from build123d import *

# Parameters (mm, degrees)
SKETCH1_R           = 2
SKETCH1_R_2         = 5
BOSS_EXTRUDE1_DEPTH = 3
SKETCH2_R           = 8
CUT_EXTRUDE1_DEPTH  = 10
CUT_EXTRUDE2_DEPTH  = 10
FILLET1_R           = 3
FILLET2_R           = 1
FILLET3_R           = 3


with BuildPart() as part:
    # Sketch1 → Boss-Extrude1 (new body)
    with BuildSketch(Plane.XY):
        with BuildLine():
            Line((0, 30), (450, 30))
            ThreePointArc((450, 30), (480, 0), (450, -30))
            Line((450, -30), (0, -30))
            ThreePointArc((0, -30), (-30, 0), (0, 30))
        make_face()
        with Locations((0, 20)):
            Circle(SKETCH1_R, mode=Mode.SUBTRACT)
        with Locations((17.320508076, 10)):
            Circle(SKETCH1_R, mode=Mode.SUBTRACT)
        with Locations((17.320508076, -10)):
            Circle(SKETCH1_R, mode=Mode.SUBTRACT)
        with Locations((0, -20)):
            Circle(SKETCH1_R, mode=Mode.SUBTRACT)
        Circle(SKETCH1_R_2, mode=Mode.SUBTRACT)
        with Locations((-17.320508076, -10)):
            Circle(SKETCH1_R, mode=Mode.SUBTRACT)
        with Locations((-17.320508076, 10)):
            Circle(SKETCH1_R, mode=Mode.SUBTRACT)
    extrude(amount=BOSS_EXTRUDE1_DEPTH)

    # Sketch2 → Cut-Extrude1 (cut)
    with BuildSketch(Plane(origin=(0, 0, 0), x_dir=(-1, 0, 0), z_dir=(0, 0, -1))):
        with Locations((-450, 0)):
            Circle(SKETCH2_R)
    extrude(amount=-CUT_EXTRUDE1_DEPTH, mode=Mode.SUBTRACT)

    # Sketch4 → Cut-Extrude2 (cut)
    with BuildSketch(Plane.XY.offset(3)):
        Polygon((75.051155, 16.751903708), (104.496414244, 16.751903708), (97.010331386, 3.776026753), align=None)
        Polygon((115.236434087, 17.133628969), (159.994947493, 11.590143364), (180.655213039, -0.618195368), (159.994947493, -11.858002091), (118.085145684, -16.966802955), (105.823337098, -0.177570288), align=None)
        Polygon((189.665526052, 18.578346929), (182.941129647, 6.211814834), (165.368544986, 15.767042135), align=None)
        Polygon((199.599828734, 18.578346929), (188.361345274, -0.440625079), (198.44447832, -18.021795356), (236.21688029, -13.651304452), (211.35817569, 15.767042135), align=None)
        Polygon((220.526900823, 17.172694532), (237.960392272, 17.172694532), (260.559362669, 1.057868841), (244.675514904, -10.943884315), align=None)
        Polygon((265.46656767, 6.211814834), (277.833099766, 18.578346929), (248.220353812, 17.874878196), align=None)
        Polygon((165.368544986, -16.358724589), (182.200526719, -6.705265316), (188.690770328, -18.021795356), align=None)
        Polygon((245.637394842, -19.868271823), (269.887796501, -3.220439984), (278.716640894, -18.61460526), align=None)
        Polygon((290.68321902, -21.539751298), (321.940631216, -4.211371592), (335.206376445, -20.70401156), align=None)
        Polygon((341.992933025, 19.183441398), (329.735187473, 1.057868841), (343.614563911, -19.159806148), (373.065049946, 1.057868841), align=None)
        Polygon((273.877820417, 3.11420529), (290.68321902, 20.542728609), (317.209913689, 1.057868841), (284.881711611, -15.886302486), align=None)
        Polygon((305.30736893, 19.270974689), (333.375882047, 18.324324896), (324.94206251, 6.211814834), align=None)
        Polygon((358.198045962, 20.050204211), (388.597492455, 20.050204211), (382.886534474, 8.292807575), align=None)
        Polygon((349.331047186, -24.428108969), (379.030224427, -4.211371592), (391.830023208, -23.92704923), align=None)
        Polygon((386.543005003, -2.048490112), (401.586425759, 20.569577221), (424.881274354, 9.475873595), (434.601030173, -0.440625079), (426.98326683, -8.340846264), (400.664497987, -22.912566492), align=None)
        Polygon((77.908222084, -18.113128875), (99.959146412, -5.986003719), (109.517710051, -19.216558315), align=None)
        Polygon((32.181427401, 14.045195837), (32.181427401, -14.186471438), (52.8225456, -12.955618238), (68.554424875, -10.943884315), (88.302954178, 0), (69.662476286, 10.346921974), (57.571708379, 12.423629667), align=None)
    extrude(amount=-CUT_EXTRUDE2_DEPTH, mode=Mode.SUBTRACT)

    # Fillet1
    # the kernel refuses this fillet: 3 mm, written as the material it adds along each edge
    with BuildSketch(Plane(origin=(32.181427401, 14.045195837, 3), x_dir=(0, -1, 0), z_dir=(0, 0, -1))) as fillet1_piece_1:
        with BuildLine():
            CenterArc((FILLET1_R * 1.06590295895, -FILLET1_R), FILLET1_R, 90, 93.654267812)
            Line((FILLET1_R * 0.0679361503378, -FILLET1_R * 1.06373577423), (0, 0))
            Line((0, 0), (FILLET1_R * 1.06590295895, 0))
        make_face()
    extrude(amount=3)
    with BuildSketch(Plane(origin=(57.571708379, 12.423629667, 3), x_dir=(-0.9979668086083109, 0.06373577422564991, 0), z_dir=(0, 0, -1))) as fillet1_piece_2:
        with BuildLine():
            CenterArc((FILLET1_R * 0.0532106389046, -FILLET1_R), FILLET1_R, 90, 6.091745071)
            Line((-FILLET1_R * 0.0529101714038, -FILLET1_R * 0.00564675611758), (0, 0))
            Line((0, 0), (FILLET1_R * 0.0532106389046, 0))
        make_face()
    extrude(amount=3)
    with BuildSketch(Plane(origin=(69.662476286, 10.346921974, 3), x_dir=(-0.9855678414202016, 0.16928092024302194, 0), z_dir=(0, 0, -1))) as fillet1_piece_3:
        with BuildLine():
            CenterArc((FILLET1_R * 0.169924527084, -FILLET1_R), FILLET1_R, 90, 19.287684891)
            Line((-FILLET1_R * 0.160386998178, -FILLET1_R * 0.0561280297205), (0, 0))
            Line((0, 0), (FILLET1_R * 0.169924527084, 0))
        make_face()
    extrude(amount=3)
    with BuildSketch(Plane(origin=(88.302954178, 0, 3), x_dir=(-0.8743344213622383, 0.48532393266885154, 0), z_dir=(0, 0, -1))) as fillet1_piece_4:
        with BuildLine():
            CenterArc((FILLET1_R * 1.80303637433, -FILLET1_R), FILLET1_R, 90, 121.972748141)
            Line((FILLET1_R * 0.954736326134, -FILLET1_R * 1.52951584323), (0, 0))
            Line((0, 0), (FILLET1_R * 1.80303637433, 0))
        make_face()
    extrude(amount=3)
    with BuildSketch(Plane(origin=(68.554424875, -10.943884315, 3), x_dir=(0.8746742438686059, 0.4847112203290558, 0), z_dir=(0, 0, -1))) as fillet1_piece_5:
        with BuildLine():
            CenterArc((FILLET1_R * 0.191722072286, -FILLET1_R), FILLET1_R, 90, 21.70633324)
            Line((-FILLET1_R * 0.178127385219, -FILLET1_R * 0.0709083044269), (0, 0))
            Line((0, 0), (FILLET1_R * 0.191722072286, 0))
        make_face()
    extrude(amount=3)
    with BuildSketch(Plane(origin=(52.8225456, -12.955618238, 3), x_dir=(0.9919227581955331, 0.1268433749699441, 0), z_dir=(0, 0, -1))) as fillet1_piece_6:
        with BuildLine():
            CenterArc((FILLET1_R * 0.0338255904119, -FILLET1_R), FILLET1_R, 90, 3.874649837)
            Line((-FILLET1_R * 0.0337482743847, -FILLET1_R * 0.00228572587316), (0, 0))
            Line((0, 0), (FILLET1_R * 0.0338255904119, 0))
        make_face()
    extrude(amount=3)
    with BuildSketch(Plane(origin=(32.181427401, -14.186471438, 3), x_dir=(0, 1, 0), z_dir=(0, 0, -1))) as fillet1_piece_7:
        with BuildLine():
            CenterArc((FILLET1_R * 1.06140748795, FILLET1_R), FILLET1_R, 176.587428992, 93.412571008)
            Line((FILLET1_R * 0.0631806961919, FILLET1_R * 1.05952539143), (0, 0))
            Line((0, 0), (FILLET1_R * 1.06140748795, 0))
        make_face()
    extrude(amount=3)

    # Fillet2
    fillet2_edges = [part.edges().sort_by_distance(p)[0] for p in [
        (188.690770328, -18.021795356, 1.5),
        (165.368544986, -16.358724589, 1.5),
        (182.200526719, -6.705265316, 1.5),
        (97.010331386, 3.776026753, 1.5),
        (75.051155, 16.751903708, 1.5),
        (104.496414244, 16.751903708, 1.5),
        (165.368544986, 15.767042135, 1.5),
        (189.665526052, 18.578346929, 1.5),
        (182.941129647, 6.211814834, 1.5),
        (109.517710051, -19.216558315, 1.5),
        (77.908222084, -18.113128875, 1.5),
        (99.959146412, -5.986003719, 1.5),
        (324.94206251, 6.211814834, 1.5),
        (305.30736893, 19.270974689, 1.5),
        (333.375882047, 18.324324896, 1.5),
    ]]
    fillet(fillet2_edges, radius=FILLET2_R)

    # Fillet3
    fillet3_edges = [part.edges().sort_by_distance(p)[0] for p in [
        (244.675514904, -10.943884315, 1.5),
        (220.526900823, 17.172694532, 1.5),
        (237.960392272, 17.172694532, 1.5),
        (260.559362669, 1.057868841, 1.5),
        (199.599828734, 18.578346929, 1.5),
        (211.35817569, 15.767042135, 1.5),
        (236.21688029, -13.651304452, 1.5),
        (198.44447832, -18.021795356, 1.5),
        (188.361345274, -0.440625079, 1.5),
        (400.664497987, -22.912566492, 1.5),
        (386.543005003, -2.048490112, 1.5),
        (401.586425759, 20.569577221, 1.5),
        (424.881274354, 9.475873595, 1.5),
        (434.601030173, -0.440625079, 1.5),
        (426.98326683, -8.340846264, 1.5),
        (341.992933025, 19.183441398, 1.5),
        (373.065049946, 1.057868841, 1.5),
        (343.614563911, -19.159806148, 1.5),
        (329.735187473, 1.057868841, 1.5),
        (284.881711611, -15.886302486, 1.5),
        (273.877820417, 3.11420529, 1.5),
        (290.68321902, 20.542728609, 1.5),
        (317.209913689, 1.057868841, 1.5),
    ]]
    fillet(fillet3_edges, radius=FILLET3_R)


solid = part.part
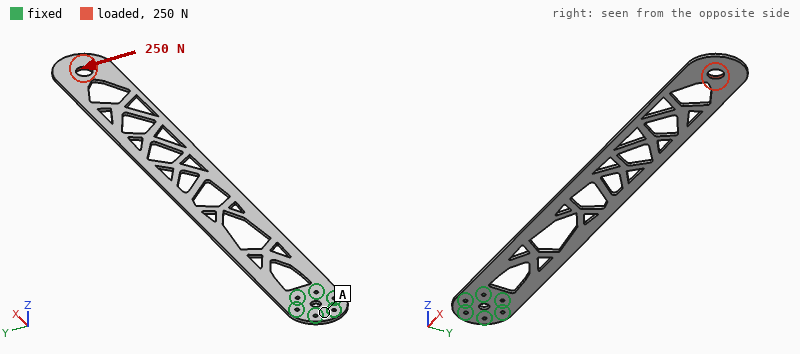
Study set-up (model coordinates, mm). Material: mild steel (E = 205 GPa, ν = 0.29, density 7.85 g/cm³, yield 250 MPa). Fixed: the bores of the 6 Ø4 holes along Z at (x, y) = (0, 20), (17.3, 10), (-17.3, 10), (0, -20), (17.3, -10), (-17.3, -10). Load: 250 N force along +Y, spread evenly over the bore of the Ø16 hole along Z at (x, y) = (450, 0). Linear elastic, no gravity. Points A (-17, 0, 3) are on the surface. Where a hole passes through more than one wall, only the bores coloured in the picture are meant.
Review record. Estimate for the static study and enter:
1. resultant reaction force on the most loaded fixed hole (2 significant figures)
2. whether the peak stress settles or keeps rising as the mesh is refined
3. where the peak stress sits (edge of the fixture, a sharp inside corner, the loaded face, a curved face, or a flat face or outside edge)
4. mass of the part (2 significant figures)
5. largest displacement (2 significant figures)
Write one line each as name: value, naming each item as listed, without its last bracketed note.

resultant reaction force on the most loaded fixed hole: 1.4 kN
whether the peak stress settles or keeps rising as the mesh is refined: keeps rising
where the peak stress sits: edge of the fixture
mass of the part: 470 g
largest displacement: 0.89 mm
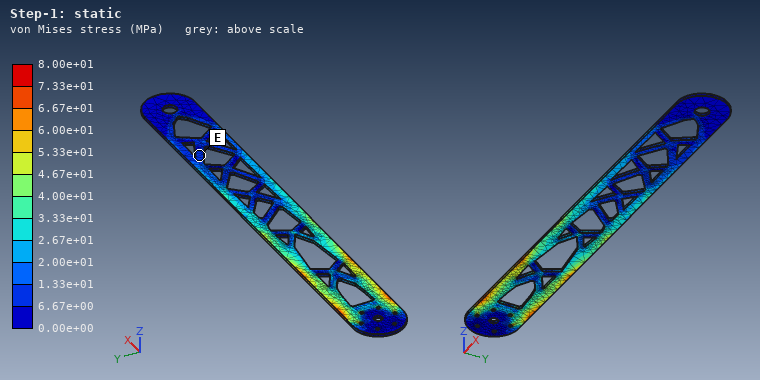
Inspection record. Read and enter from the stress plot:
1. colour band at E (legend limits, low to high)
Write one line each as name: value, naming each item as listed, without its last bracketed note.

colour band at E: 6.67e+00 to 1.33e+01 MPa
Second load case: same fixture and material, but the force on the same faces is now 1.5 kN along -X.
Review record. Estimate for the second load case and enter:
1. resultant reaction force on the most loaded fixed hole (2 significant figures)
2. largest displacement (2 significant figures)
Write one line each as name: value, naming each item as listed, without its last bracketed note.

resultant reaction force on the most loaded fixed hole: 390 N
largest displacement: 46 µm
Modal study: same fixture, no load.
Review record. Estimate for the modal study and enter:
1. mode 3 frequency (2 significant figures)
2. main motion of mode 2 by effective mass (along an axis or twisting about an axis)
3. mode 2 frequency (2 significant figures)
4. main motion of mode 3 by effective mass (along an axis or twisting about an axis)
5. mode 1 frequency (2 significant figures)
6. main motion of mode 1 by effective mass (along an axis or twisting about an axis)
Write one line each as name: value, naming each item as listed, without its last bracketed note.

mode 3 frequency: 140 Hz
main motion of mode 2 by effective mass: along Z
mode 2 frequency: 67 Hz
main motion of mode 3 by effective mass: twisting about X
mode 1 frequency: 11 Hz
main motion of mode 1 by effective mass: along Z
